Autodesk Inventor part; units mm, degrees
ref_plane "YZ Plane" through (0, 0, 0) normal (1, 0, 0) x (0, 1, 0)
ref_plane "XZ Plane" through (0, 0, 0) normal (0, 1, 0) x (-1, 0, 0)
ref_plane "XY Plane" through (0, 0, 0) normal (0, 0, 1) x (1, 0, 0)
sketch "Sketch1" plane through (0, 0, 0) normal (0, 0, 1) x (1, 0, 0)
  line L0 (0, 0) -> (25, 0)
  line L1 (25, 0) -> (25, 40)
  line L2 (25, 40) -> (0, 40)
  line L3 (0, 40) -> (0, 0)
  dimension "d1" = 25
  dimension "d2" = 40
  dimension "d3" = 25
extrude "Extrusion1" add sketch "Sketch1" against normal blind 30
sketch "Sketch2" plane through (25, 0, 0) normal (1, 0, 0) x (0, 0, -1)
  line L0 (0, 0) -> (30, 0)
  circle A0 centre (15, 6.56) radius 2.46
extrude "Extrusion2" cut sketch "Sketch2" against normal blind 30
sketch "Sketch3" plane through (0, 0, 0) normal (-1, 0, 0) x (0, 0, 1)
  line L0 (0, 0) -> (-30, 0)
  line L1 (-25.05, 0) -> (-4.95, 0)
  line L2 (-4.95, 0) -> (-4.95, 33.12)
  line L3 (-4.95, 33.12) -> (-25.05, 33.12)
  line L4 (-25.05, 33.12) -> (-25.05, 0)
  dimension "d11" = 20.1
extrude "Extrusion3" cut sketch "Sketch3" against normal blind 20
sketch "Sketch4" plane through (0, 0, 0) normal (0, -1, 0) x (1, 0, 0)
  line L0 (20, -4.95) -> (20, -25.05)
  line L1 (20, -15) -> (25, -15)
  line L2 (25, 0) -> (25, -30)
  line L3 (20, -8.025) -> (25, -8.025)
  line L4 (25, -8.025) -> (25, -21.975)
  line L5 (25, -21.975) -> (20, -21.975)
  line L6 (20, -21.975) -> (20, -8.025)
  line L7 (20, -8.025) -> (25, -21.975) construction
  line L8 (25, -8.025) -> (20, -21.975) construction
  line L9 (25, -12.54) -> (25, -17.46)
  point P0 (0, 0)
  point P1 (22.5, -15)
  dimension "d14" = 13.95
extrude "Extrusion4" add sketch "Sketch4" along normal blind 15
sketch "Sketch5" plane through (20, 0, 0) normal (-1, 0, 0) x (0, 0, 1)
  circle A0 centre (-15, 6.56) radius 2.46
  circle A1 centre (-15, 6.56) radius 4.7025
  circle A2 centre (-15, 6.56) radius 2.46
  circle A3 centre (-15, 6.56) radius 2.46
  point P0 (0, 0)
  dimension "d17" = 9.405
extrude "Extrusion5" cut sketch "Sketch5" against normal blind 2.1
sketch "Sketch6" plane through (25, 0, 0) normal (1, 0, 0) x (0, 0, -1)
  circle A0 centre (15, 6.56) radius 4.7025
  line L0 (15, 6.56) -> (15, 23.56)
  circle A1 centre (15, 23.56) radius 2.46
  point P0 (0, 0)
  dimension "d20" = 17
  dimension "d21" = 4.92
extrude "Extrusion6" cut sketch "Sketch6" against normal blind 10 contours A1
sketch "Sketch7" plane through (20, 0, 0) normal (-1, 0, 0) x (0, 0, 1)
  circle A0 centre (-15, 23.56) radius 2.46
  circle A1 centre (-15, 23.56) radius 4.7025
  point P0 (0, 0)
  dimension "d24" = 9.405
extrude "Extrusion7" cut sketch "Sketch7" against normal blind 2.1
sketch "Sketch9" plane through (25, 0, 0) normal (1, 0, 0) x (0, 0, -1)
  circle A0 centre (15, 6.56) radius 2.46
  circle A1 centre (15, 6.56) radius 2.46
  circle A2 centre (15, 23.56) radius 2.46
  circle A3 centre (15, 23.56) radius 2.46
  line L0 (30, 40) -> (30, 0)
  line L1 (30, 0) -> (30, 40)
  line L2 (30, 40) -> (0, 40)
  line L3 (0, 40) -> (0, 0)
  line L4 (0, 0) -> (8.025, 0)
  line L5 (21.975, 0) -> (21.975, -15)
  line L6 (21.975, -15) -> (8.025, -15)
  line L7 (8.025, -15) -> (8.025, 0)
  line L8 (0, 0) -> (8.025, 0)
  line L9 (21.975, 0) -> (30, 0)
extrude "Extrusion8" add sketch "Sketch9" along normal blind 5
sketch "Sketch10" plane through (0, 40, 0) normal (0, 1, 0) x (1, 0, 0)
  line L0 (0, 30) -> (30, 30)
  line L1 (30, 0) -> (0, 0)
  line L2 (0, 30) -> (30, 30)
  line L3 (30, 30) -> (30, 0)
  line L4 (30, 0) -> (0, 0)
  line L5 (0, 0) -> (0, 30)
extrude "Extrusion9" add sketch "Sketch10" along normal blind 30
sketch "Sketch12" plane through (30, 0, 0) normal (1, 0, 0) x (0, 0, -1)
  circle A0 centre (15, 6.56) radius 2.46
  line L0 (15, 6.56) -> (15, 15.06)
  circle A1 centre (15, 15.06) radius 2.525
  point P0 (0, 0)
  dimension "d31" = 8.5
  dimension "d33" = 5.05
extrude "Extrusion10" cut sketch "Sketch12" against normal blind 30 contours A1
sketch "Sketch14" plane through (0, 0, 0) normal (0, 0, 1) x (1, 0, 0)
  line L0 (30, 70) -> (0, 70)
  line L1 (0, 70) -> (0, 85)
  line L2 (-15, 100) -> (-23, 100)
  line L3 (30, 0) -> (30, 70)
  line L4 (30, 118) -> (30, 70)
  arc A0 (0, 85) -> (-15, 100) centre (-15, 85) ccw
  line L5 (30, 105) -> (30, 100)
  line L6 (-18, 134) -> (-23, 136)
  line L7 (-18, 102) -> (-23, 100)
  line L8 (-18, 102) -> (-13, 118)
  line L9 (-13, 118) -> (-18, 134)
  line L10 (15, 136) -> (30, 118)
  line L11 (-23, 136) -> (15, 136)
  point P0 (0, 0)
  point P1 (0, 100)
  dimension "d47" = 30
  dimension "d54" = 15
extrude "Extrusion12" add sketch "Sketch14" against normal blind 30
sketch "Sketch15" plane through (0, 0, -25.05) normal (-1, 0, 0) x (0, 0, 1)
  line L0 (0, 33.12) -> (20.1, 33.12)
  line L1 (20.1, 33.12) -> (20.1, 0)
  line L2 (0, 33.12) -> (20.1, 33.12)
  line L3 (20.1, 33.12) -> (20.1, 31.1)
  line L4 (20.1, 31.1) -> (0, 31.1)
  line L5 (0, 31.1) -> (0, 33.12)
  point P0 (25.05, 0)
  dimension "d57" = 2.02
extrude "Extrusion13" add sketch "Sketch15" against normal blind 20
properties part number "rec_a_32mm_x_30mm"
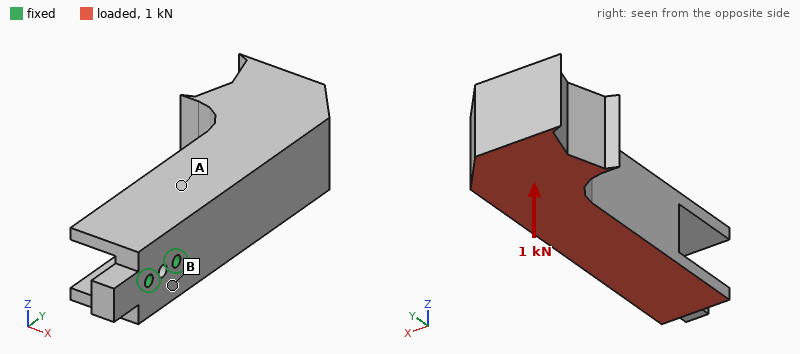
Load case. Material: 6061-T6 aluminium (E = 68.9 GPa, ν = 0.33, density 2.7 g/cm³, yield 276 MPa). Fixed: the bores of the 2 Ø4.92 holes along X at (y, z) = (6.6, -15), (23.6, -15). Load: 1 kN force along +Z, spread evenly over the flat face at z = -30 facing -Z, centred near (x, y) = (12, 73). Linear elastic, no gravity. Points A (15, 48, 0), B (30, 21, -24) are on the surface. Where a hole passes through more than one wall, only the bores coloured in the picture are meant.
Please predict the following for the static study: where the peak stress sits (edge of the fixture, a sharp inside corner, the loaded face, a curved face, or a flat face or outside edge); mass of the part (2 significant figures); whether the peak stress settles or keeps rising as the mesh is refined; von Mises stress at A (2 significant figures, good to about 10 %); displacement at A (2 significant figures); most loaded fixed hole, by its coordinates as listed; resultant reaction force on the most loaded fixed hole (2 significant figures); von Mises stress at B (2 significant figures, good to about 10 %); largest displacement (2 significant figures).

edge of the fixture
340 g
keeps rising
7.5 MPa
0.029 mm
(23.6, -15)
3.1 kN
17 MPa
0.14 mm
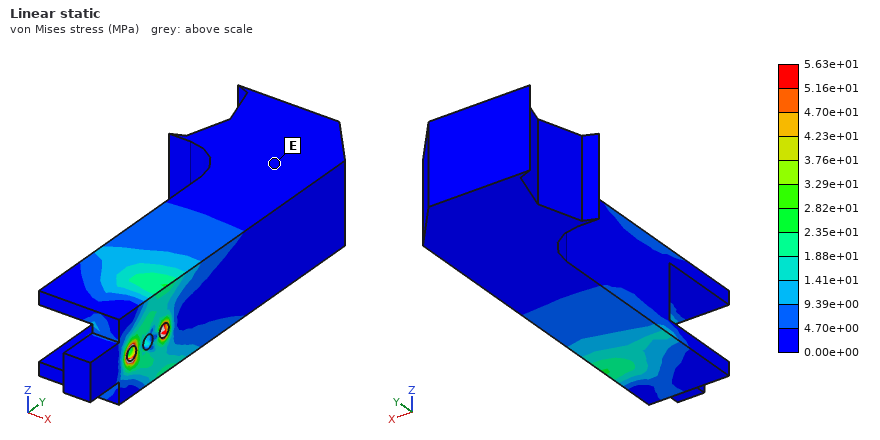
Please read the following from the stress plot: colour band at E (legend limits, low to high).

0.00e+00 to 4.70e+00 MPa
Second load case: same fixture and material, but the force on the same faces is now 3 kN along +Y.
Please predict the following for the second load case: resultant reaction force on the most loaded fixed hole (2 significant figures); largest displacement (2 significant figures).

3.1 kN
0.16 mm
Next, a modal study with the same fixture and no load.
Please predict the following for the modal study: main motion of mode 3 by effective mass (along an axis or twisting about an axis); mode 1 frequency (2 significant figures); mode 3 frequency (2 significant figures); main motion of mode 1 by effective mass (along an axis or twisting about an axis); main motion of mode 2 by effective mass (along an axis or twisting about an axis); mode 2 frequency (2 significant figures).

twisting about Y
770 Hz
2600 Hz
along X
along Z
900 Hz
